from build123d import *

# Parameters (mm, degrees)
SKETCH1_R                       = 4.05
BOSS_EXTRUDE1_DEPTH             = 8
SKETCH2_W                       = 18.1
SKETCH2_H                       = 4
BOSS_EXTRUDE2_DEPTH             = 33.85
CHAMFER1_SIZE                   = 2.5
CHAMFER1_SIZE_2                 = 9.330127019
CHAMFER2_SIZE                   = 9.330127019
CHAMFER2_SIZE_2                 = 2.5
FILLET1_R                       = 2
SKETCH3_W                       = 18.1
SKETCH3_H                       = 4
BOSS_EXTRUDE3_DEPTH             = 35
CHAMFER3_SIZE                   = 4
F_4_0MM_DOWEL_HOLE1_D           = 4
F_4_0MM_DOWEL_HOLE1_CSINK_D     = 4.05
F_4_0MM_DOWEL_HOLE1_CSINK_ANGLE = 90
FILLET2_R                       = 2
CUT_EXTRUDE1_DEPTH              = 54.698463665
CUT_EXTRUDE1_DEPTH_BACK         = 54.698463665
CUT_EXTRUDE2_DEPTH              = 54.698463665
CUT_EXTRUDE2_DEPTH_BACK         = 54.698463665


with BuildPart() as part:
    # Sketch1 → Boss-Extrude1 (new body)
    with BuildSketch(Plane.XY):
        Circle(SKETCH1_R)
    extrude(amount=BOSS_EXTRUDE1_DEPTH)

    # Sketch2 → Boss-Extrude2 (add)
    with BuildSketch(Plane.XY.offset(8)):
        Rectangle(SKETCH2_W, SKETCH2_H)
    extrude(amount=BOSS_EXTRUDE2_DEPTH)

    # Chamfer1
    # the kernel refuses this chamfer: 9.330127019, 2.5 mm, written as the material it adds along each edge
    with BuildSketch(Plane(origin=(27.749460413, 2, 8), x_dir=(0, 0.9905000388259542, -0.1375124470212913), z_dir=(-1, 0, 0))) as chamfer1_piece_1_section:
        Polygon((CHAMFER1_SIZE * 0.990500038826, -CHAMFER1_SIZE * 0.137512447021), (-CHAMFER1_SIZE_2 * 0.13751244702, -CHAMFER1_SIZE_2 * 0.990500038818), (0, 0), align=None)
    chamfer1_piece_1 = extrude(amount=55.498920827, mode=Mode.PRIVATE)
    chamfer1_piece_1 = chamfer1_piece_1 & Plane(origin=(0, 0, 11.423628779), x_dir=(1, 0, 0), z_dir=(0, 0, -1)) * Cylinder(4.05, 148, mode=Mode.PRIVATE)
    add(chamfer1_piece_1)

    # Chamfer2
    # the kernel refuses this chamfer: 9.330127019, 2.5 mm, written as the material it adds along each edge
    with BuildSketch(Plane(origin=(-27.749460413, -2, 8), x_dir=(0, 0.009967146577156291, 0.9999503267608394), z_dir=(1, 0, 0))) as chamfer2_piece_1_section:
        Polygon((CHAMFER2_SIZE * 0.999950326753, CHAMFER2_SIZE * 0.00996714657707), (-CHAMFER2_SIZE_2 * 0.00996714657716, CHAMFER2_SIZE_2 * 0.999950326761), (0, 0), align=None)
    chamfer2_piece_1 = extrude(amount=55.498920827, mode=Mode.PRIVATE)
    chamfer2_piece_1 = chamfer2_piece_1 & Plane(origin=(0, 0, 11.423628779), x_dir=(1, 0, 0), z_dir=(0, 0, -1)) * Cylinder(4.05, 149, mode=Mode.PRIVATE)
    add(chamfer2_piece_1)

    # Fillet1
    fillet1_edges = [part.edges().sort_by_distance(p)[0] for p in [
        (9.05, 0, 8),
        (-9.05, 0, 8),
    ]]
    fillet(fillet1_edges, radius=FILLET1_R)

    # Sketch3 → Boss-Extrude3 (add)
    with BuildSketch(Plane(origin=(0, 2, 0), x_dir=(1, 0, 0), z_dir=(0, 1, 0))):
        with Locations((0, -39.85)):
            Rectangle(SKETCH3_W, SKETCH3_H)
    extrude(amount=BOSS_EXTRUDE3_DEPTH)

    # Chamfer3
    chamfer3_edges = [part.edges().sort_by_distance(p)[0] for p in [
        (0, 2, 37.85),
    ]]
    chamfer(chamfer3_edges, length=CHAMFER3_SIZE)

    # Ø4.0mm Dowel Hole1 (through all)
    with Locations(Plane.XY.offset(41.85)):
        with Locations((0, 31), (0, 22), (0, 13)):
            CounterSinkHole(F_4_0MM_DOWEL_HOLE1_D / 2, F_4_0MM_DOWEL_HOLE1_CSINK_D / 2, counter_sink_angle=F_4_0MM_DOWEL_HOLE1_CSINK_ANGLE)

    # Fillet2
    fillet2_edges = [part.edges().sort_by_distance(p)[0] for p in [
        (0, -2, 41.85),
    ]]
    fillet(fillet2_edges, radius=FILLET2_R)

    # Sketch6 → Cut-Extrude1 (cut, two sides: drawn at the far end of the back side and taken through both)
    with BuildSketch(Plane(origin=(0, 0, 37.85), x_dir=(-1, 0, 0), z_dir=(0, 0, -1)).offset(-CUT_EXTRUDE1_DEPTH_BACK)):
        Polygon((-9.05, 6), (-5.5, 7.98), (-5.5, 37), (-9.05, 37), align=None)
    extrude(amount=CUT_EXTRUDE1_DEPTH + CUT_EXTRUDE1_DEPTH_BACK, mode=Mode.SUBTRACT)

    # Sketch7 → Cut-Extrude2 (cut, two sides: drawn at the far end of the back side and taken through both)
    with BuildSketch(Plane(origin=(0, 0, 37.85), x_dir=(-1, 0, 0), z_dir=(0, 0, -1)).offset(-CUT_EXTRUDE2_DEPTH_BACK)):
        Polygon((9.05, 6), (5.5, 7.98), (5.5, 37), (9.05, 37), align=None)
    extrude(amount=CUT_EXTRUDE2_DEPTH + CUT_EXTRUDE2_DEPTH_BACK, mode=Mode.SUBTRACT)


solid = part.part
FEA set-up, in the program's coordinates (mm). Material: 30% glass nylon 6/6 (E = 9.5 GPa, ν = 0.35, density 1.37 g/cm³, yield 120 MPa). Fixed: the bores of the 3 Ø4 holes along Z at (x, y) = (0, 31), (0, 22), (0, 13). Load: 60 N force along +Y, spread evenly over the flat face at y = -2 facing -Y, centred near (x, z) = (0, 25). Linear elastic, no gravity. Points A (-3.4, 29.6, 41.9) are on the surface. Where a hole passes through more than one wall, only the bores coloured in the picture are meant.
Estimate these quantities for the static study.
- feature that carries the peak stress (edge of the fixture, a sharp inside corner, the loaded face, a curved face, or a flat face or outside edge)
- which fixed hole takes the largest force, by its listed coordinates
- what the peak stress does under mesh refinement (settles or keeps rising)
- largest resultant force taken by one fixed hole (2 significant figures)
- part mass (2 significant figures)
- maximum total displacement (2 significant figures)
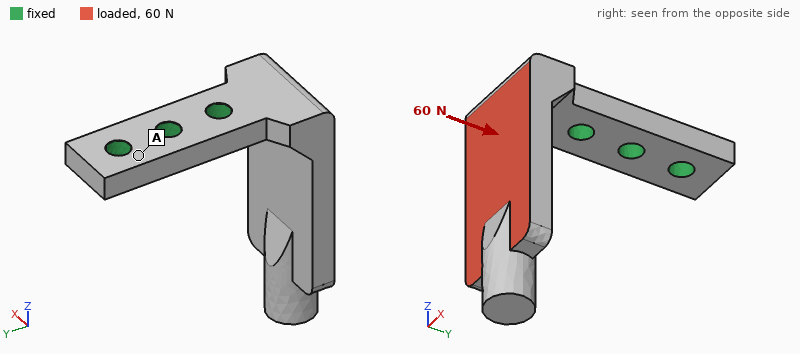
edge of the fixture
(0, 13)
keeps rising
56 N
6.4 g
0.65 mm
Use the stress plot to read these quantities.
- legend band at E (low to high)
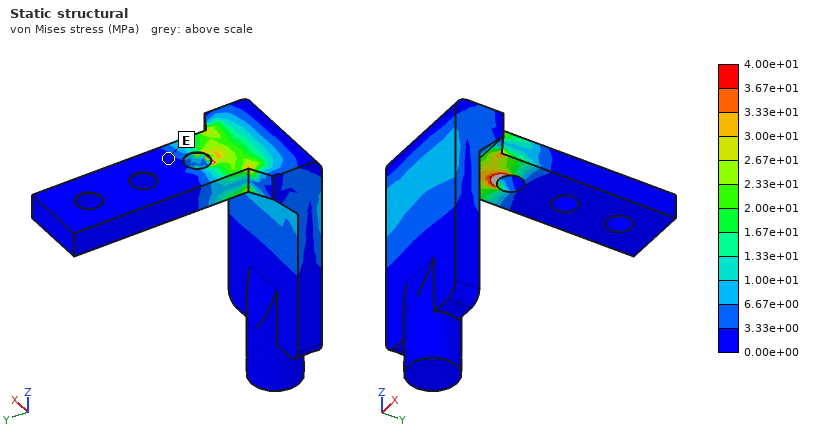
0.00e+00 to 3.33e+00 MPa
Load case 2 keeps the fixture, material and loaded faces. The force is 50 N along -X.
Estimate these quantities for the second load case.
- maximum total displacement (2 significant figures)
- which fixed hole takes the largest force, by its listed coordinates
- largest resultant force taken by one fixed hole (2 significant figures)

0.28 mm
(0, 13)
79 N
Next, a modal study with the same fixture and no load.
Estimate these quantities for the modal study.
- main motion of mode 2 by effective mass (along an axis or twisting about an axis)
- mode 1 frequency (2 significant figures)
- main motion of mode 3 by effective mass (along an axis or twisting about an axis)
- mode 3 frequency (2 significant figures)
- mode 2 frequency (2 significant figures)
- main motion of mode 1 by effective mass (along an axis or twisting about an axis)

along X
790 Hz
along Z
3400 Hz
1100 Hz
along Y
